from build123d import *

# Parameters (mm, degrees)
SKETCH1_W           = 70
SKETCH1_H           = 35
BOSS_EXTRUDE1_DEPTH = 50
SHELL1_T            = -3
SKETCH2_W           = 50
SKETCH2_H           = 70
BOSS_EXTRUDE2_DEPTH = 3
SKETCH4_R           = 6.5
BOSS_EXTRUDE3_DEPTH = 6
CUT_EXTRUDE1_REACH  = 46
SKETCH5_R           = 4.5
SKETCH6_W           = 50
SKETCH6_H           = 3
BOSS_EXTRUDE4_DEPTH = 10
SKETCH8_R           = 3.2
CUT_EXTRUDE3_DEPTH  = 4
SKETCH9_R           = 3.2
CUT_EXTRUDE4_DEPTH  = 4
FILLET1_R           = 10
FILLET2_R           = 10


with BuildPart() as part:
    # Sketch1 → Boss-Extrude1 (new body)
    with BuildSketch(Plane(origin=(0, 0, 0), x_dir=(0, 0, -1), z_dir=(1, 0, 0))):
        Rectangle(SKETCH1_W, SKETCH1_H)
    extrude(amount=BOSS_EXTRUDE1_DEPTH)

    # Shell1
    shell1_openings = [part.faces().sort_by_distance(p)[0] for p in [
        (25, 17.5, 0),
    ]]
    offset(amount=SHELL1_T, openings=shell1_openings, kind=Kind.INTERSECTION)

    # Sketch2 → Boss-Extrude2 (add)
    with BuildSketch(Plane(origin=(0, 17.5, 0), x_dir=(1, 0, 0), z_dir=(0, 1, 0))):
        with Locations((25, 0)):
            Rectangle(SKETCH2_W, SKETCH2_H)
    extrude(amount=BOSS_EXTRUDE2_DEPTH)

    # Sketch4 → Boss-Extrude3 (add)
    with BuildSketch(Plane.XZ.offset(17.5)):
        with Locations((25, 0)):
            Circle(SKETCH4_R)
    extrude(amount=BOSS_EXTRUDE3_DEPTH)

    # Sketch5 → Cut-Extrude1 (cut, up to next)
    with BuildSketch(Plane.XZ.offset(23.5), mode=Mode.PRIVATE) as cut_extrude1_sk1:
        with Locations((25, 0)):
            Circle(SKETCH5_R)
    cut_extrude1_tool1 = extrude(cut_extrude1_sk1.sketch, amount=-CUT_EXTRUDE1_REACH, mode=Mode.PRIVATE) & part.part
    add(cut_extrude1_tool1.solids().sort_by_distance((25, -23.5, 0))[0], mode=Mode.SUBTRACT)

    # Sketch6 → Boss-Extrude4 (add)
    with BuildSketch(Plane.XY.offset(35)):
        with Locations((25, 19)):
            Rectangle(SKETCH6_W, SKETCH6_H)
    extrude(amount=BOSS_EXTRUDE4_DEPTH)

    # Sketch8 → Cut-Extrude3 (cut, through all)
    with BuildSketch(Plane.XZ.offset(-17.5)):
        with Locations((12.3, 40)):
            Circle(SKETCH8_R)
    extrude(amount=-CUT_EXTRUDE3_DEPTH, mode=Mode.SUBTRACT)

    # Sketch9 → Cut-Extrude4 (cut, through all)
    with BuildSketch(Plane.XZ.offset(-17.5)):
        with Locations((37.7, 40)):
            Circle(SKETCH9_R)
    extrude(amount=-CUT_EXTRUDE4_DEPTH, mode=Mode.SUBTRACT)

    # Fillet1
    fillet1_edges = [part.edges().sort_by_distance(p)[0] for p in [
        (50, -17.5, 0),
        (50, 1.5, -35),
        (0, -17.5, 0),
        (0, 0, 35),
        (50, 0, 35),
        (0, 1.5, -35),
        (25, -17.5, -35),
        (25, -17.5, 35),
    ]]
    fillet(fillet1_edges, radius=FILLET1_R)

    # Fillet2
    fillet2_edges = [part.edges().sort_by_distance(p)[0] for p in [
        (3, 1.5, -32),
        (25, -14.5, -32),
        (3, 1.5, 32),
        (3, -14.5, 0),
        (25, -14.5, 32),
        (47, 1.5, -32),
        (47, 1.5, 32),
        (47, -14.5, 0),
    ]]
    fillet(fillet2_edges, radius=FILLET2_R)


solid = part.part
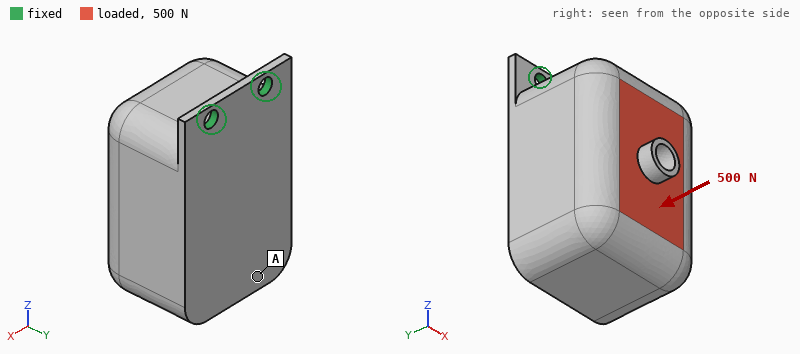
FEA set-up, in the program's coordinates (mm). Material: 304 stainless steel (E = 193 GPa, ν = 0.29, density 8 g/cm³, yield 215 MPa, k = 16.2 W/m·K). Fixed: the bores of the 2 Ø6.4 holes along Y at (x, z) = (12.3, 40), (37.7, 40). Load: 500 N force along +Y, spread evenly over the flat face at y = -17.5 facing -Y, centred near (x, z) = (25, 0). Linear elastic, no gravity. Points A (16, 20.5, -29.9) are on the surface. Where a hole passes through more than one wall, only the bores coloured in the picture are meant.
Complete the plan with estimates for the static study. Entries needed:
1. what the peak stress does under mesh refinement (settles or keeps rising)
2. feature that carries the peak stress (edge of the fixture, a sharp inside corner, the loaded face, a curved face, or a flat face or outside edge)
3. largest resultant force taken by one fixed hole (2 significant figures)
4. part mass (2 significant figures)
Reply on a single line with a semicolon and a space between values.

keeps rising; edge of the fixture; 260 N; 350 g
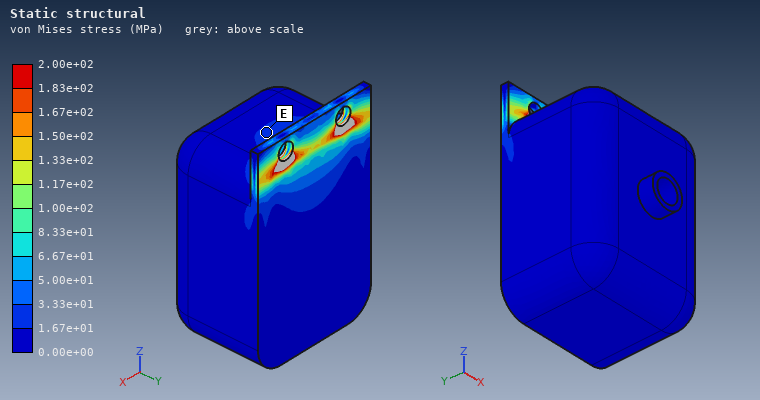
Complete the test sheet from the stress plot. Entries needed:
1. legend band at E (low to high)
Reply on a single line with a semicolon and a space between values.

1.67e+01 to 3.33e+01 MPa
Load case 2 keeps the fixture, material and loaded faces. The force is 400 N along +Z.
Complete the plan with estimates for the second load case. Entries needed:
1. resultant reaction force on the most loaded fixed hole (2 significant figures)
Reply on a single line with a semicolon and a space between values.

200 N
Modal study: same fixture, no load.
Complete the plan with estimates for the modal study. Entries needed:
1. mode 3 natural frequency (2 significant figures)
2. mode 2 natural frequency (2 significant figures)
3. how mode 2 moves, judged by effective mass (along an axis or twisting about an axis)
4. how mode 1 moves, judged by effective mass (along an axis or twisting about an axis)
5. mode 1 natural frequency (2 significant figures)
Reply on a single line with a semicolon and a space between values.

3300 Hz; 2200 Hz; along X; along Y; 320 Hz
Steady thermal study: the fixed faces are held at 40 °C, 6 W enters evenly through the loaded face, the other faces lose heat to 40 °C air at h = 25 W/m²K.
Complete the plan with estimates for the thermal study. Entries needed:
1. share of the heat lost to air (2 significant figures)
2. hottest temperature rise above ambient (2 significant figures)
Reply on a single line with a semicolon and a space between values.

86 %; 21 K
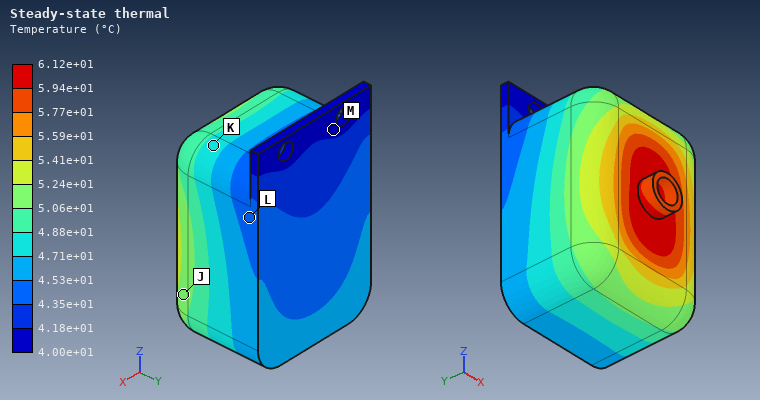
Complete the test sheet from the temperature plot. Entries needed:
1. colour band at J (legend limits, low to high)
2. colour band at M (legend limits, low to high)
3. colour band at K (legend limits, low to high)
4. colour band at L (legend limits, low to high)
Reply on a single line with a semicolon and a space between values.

5.06e+01 to 5.24e+01 °C; 4.00e+01 to 4.18e+01 °C; 4.71e+01 to 4.88e+01 °C; 4.35e+01 to 4.53e+01 °C
